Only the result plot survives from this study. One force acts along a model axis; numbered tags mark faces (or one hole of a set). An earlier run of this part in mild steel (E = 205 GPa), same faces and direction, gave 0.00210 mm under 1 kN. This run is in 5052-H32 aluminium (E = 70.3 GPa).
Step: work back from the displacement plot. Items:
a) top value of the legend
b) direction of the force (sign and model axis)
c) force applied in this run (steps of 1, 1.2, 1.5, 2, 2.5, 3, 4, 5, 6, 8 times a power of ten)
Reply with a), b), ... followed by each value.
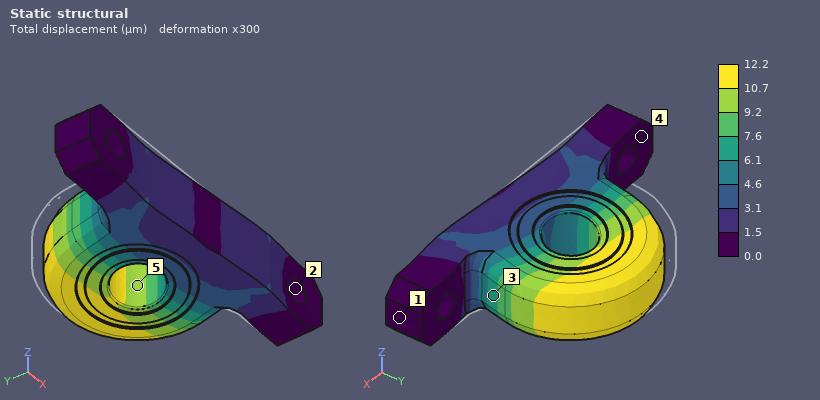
a) 12.2 µm
b) +X
c) 2 kN
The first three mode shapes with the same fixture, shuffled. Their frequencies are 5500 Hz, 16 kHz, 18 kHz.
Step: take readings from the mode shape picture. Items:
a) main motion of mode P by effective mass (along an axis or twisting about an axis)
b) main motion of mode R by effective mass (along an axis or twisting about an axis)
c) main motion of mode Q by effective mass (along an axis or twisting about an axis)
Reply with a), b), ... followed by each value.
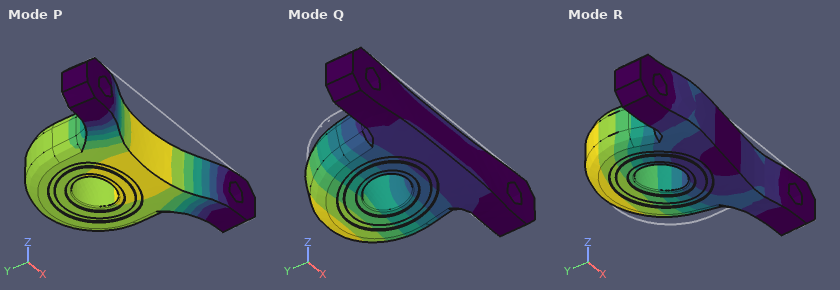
a) along Y
b) along X
c) along Z
